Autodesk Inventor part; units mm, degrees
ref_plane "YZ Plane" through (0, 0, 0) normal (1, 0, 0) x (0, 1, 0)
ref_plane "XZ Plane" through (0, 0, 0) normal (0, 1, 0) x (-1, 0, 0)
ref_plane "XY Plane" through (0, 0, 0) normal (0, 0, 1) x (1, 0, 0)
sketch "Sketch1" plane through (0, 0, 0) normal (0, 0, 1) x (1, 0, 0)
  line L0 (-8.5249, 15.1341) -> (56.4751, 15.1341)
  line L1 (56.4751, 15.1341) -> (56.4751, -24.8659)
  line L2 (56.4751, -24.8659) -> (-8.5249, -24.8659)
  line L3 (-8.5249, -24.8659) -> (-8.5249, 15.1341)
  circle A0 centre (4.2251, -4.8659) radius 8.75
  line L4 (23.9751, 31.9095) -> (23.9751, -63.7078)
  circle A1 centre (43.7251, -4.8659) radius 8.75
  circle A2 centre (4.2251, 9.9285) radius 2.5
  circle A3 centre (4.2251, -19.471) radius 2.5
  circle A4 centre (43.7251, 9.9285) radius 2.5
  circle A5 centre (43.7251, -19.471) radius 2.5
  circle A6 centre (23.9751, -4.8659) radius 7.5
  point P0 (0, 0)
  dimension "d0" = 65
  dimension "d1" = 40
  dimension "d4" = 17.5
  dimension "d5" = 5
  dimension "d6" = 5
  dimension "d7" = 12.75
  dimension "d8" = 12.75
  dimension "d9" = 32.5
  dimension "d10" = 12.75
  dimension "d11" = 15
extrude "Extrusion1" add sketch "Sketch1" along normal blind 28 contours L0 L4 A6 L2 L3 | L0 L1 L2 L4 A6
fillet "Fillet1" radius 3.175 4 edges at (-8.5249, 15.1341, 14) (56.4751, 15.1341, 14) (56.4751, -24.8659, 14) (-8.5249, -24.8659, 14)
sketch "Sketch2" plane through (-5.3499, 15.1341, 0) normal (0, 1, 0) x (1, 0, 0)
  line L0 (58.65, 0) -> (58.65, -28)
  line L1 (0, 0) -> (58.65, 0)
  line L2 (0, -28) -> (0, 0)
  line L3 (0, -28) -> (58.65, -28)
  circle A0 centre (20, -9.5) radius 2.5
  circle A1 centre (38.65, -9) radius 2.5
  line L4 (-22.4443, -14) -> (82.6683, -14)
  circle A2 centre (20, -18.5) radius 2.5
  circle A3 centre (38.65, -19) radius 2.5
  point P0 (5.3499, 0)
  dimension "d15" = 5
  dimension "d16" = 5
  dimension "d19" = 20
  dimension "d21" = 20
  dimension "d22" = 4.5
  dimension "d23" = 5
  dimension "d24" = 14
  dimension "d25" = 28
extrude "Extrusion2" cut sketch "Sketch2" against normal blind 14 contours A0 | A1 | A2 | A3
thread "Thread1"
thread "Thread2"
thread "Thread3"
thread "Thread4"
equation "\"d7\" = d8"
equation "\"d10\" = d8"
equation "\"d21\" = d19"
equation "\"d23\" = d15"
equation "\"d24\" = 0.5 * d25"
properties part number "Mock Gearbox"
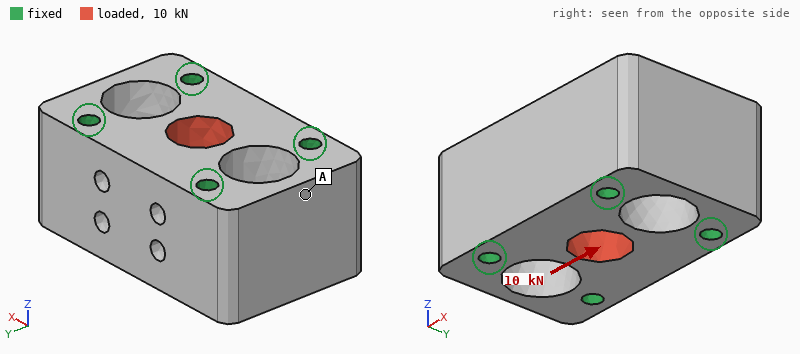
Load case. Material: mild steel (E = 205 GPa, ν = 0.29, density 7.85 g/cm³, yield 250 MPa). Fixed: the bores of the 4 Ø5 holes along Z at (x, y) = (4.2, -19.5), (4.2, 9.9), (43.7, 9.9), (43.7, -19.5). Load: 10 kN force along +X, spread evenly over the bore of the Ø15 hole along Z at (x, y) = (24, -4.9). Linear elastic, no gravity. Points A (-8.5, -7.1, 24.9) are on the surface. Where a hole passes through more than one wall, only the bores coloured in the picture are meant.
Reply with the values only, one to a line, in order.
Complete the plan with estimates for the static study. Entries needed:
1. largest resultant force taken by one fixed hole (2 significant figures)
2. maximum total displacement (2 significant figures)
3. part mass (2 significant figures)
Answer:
2.8 kN
1.4 µm
400 g
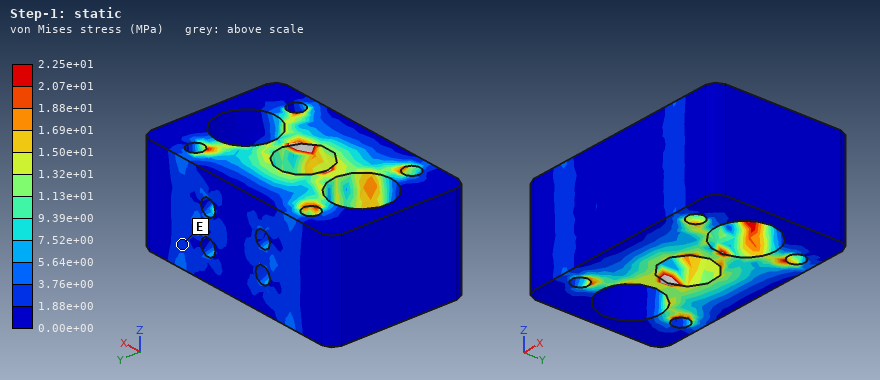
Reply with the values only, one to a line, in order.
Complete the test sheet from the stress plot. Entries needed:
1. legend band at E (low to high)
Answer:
1.88e+00 to 3.76e+00 MPa
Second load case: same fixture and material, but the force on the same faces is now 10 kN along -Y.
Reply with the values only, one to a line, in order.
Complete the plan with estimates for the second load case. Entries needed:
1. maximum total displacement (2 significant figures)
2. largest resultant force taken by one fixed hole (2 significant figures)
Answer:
2.3 µm
2.9 kN
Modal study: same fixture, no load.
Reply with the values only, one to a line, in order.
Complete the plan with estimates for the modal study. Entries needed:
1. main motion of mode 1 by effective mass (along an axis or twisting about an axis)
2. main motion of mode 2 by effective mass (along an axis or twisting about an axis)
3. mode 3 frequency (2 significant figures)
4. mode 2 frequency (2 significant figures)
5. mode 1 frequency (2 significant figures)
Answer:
along Y
along Z
35 kHz
32 kHz
29 kHz
